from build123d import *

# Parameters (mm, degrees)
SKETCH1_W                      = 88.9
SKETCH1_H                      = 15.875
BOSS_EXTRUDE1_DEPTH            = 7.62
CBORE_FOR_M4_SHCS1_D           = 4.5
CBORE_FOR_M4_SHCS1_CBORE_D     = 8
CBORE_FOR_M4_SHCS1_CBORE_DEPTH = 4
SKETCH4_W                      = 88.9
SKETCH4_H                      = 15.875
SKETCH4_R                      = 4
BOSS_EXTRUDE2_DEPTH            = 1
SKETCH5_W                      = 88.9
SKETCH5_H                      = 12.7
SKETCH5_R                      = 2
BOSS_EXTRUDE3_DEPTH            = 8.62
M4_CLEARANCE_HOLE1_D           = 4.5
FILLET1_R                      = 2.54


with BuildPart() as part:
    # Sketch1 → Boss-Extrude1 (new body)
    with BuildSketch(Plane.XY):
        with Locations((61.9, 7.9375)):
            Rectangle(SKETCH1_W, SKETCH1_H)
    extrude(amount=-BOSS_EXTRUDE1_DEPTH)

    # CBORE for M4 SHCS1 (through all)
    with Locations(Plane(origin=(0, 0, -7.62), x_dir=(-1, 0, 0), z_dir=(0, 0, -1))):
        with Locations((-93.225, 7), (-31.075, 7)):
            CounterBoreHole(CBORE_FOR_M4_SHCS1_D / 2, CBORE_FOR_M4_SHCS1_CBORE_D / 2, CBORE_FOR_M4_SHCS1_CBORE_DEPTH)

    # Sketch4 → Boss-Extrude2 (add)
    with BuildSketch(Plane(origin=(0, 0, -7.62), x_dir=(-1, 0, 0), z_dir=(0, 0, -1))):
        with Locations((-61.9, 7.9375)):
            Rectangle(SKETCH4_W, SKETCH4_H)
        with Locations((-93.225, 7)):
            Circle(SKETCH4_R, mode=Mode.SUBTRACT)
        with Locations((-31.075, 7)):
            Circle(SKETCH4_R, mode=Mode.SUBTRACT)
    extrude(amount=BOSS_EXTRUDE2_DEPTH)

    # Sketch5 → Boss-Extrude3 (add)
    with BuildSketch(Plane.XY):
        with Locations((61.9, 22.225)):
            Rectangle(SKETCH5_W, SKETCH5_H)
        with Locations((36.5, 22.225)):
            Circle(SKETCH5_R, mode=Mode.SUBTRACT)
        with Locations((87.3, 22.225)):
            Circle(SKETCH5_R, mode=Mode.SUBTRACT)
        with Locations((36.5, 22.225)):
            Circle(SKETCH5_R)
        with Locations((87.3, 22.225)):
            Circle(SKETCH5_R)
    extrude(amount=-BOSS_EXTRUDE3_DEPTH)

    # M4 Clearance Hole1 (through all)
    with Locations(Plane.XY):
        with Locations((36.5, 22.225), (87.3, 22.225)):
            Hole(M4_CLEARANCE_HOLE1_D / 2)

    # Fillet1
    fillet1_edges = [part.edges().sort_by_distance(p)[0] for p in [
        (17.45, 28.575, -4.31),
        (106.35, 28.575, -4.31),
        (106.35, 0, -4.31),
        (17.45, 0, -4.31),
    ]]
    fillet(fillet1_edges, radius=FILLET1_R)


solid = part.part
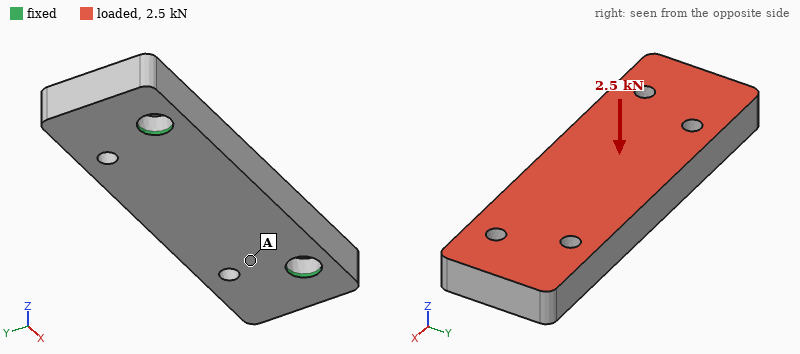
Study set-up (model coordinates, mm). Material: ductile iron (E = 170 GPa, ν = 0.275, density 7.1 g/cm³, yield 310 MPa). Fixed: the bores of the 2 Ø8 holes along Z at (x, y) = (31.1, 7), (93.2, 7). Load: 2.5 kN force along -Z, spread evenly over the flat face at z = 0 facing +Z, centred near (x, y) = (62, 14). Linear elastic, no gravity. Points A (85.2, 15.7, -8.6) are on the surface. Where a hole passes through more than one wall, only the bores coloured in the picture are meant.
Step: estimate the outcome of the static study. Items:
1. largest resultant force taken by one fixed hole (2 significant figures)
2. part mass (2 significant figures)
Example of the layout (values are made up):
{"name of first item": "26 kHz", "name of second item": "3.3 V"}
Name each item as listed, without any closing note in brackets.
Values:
{"largest resultant force taken by one fixed hole": "1.4 kN", "part mass": "150 g"}
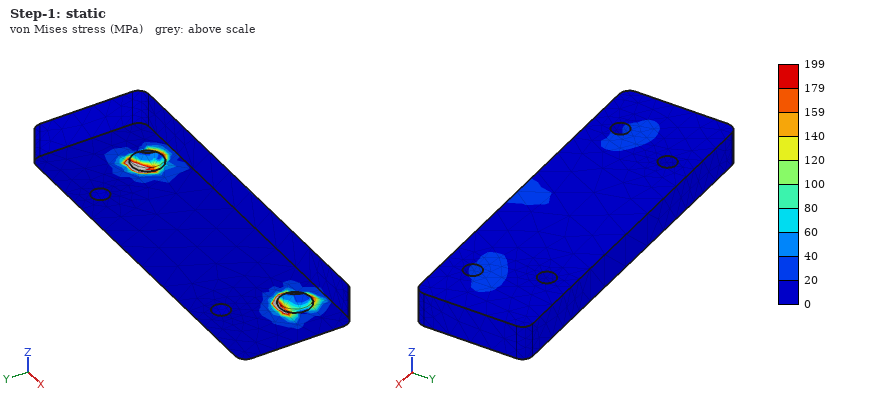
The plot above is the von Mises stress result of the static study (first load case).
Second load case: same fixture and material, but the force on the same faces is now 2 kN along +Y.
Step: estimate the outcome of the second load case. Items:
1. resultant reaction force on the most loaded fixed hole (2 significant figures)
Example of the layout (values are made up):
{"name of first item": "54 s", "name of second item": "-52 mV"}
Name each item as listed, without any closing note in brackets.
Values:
{"resultant reaction force on the most loaded fixed hole": "1.0 kN"}
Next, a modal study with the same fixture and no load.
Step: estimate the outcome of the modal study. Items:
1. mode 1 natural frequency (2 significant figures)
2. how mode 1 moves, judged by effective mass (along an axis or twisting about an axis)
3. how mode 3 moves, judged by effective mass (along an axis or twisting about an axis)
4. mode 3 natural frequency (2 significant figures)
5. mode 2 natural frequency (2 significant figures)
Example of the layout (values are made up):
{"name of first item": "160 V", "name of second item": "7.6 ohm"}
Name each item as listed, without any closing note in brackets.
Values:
{"mode 1 natural frequency": "4700 Hz", "how mode 1 moves, judged by effective mass": "along Z", "how mode 3 moves, judged by effective mass": "twisting about Y", "mode 3 natural frequency": "8900 Hz", "mode 2 natural frequency": "8400 Hz"}
